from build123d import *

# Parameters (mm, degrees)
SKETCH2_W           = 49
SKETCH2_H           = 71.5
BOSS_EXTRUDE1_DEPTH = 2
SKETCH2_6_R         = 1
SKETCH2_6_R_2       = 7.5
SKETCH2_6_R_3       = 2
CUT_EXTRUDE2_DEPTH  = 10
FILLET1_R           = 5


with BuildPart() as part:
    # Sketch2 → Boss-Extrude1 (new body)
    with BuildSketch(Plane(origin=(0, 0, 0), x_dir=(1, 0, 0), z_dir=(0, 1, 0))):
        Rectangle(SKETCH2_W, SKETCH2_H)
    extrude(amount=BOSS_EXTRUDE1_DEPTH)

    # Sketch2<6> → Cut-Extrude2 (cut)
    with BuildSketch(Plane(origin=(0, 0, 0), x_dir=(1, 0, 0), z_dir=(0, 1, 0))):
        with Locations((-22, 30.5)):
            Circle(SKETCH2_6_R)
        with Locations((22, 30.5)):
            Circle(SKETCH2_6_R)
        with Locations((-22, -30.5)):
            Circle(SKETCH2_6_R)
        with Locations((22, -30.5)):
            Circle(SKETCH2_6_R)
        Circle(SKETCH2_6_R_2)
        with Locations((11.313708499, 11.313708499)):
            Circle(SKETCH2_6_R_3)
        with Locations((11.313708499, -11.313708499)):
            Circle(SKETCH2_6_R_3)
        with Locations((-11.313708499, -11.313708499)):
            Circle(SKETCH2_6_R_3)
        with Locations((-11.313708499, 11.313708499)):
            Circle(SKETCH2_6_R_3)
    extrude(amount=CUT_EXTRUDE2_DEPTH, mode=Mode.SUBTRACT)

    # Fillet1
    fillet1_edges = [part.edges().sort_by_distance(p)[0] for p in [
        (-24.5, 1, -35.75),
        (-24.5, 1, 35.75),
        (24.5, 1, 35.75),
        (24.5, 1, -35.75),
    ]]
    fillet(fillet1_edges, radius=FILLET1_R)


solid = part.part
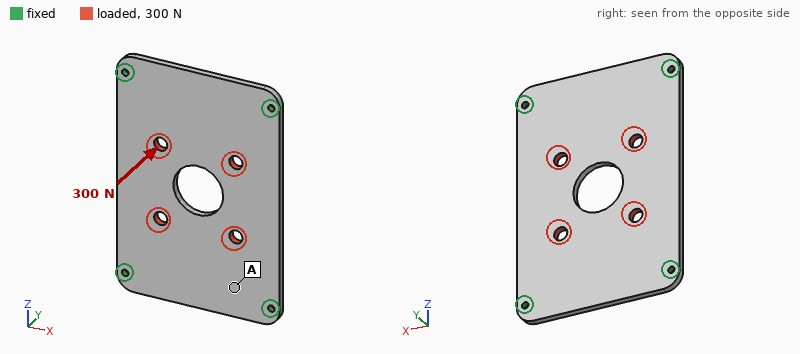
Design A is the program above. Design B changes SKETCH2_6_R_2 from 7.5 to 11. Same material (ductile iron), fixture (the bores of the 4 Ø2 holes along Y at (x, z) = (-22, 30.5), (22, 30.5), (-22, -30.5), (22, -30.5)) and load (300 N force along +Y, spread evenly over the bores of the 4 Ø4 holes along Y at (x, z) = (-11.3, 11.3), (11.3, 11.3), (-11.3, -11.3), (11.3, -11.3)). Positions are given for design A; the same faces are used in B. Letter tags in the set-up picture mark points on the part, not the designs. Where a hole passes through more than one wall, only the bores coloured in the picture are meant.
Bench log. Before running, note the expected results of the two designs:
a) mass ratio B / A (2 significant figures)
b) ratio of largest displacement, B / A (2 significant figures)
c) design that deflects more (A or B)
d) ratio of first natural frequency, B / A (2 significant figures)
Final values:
0.94
1.1
B
1.0
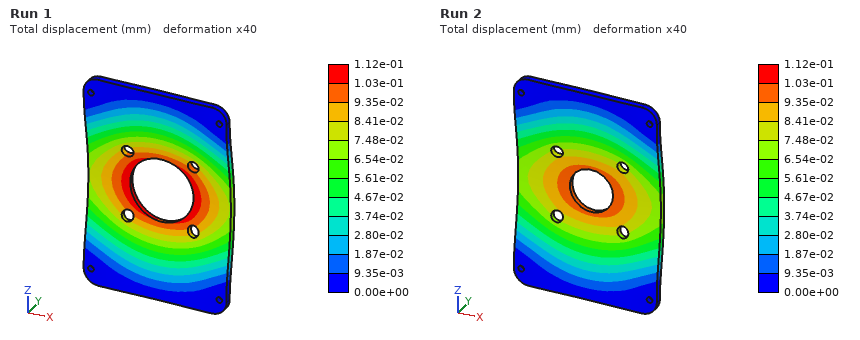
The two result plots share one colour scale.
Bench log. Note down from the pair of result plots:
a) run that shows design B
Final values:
Run 1
